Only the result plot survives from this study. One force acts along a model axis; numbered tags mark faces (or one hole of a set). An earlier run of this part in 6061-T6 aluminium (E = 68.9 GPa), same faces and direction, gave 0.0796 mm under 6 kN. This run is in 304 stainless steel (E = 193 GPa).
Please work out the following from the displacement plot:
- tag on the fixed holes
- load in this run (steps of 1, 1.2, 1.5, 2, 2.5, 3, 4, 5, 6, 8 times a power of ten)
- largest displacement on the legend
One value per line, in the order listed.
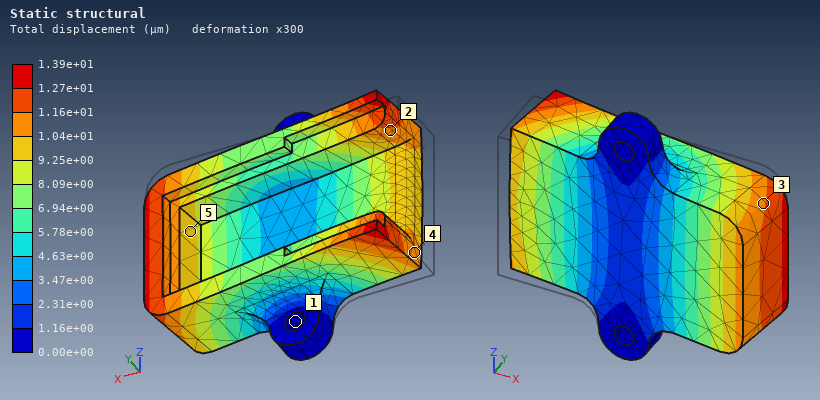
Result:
1
3 kN
1.39e+01 µm
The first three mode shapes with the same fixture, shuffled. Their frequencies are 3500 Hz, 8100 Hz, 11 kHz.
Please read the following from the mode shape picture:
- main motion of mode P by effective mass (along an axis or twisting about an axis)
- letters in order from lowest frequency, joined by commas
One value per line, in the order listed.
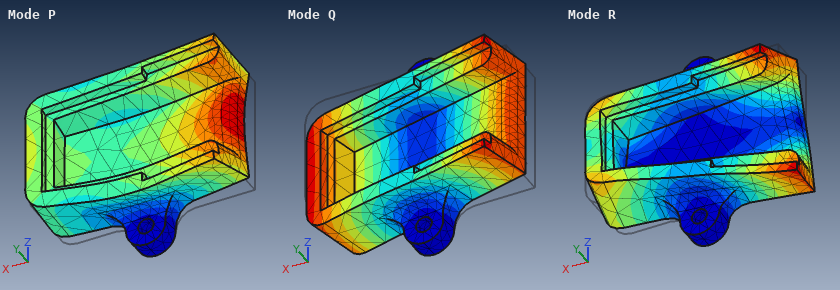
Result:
along Y
Q, P, R
